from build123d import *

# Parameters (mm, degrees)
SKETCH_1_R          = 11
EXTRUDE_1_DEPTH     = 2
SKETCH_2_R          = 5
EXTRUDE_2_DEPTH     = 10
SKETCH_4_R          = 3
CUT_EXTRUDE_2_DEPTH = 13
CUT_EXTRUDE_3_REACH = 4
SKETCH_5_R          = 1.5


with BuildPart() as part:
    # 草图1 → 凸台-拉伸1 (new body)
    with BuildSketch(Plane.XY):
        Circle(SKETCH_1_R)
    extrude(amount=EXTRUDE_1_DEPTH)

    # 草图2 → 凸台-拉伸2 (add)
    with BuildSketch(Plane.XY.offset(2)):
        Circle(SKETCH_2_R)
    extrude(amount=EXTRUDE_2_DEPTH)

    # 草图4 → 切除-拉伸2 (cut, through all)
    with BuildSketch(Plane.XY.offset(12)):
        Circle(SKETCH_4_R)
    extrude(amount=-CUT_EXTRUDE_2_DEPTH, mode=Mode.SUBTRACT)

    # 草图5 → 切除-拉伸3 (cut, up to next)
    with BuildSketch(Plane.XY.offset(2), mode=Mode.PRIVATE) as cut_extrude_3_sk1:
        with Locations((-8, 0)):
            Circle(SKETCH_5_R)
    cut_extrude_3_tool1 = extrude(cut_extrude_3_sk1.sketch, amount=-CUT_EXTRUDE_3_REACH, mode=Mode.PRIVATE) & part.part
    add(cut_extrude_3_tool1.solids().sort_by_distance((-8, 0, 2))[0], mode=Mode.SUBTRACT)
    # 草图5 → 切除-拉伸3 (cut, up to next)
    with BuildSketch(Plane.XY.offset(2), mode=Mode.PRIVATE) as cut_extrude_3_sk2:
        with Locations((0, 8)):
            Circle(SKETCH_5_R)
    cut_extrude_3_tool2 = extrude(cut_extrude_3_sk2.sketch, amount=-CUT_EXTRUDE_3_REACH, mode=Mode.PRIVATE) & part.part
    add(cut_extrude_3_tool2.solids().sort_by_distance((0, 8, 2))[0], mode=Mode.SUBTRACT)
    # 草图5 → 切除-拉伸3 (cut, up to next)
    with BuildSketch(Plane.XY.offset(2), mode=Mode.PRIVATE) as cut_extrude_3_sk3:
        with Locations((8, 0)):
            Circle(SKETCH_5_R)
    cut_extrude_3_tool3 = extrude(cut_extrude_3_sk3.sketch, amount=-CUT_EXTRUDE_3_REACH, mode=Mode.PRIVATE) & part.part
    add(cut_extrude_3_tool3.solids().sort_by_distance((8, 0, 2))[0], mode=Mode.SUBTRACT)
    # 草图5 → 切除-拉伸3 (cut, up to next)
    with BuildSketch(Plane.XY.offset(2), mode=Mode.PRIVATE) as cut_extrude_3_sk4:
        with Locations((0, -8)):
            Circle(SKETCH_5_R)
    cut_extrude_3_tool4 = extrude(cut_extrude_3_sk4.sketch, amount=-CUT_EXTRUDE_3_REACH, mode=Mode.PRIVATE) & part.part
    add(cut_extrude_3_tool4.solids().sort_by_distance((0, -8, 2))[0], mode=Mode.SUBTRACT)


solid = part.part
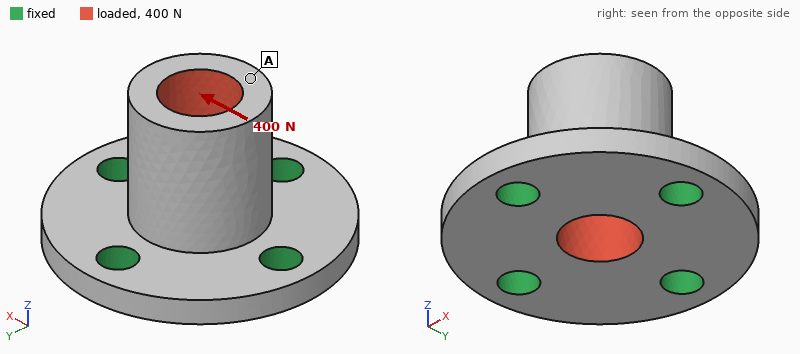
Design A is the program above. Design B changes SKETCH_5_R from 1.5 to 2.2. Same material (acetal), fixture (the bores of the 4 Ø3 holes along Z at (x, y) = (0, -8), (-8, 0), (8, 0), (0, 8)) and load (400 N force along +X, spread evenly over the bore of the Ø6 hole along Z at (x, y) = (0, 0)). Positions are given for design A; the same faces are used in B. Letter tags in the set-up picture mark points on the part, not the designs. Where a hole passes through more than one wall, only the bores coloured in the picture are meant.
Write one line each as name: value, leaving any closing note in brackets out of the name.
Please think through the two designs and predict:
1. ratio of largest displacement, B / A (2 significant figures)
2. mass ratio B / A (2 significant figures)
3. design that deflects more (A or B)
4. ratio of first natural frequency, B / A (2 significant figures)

ratio of largest displacement, B / A: 0.79
mass ratio B / A: 0.94
design that deflects more: A
ratio of first natural frequency, B / A: 1.1
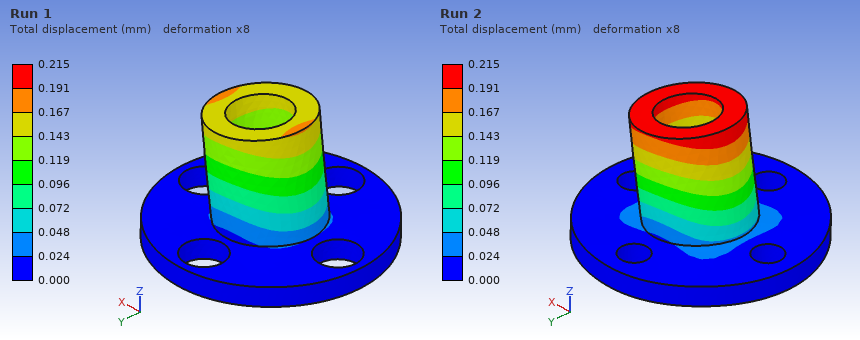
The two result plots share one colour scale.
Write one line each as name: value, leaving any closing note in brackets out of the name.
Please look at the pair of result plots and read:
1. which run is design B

which run is design B: Run 1
